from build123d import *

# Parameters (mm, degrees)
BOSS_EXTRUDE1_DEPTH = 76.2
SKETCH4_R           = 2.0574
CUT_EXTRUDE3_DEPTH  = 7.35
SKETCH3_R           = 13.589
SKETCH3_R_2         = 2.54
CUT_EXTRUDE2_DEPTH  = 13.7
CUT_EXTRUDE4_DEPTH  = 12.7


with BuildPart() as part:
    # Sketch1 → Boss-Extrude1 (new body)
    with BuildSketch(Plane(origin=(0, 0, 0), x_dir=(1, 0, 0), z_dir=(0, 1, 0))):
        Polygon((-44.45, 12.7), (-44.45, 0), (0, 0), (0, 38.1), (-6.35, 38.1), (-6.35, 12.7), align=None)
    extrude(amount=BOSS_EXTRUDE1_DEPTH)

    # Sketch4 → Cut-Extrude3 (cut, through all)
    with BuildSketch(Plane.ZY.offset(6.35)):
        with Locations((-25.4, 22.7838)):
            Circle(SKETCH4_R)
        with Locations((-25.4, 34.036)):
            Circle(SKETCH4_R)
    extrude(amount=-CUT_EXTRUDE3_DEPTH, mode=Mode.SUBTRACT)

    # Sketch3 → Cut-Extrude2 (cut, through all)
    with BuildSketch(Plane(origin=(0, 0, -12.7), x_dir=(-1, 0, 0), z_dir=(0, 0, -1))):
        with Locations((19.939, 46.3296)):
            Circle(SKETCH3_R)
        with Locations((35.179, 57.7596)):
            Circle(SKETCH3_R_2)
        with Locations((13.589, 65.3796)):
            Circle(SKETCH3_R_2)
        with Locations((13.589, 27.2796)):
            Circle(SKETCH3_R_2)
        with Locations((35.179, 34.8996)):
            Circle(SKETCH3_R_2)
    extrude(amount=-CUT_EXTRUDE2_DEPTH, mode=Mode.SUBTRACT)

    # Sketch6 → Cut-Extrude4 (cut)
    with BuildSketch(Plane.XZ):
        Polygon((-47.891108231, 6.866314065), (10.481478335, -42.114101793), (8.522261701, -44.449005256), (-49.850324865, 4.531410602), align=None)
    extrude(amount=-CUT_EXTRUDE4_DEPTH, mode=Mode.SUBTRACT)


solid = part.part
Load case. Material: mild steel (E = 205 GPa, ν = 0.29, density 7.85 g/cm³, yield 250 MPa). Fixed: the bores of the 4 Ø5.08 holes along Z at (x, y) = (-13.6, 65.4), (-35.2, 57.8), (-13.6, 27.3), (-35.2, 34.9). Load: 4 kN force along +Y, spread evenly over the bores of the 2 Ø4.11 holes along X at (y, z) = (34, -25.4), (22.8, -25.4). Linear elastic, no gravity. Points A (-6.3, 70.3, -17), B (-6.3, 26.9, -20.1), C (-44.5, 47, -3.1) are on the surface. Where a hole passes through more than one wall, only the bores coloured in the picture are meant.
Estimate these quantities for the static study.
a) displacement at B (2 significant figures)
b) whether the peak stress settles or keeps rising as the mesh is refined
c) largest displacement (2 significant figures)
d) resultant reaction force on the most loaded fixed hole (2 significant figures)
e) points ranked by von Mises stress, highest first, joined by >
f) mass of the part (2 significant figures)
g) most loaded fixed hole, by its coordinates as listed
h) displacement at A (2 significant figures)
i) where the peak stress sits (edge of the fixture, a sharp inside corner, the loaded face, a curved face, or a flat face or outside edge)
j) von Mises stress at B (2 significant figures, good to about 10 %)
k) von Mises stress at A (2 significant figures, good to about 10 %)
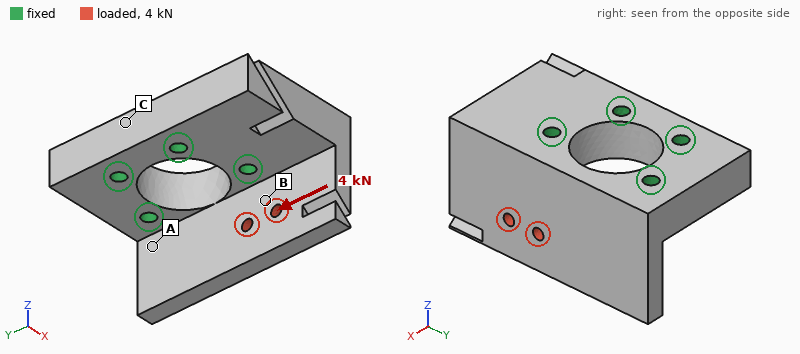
4.7 µm
keeps rising
10 µm
3.3 kN
B > A > C
360 g
(-13.6, 27.3)
3.1 µm
edge of the fixture
30 MPa
17 MPa
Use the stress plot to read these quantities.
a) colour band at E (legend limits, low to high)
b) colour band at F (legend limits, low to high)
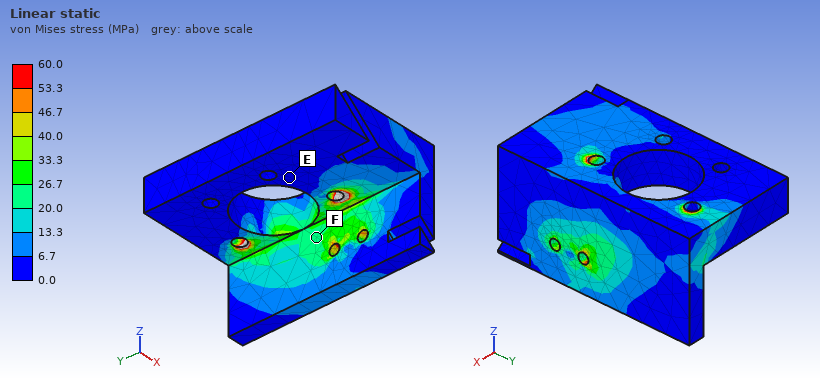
0.0 to 6.7 MPa
20.0 to 26.7 MPa
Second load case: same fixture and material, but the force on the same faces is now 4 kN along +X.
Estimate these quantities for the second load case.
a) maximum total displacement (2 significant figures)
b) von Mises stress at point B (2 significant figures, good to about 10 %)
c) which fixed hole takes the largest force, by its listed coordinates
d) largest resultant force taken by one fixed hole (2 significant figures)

71 µm
50 MPa
(-13.6, 27.3)
3.5 kN
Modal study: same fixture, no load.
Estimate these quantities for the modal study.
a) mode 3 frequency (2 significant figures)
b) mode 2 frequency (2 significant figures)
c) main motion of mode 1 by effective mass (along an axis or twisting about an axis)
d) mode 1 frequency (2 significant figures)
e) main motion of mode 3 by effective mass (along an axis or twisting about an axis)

10 kHz
7300 Hz
along X
5400 Hz
along Z
